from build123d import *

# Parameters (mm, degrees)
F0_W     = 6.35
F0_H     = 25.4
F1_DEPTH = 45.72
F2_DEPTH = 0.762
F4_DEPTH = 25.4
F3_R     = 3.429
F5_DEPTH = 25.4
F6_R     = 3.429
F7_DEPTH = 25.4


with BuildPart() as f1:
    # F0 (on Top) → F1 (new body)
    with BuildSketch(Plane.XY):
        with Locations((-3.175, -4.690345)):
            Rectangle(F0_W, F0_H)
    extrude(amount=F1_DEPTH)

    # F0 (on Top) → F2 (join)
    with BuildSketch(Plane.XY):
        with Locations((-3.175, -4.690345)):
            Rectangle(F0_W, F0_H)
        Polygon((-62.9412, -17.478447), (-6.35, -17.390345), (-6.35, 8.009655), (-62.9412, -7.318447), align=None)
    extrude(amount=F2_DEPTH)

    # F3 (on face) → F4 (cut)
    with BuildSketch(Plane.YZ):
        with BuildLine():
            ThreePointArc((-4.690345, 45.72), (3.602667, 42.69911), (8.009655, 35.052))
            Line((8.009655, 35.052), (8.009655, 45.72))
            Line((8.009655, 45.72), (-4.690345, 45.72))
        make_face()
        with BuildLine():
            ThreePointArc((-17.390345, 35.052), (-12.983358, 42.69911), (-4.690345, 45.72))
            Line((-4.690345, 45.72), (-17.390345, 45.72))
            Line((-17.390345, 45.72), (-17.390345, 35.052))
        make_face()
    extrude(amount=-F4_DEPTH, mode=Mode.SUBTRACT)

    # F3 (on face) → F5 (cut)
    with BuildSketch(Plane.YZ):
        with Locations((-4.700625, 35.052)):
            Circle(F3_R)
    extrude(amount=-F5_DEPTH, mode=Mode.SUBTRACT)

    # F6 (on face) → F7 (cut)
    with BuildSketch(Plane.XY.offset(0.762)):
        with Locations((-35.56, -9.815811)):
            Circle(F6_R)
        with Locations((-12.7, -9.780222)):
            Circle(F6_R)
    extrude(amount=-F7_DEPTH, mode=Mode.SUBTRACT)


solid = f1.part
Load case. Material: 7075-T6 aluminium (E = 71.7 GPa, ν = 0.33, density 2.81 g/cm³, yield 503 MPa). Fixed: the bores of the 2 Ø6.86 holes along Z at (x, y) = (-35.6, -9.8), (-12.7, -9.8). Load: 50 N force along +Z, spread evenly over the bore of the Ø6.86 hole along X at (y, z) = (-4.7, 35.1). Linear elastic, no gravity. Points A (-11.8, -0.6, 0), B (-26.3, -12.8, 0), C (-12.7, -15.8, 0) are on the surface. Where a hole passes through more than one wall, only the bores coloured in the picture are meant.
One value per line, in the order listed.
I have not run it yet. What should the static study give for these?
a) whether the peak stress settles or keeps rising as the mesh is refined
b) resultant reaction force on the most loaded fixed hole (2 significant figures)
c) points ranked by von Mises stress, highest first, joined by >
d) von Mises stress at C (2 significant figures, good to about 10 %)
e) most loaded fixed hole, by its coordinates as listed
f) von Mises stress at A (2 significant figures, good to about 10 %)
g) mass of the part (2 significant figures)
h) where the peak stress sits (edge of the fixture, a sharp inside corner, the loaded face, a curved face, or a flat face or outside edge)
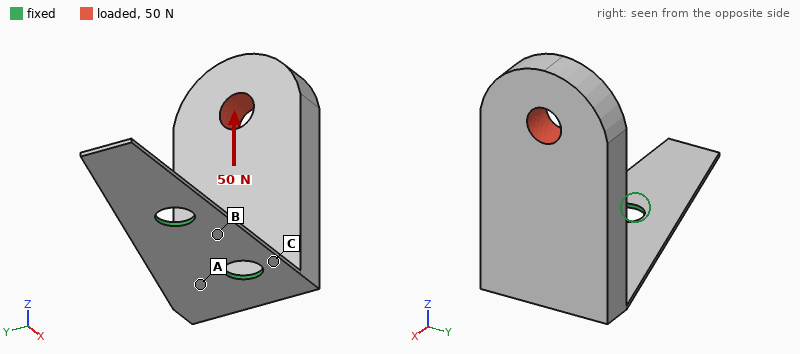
keeps rising
51 N
A > C > B
30 MPa
(-12.7, -9.8)
48 MPa
21 g
edge of the fixture
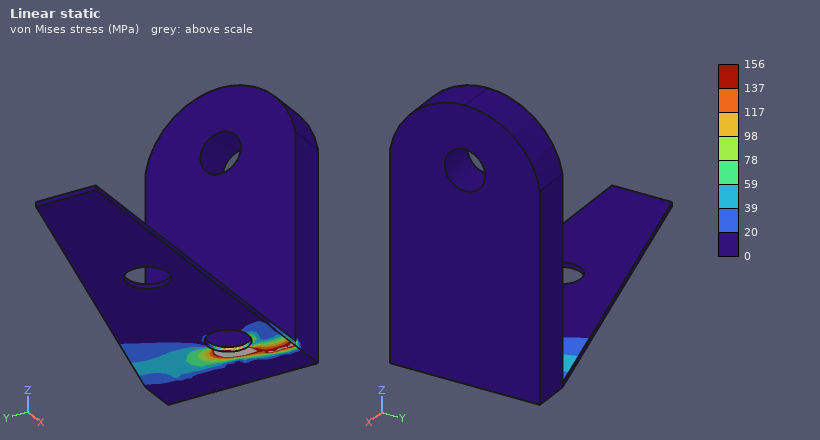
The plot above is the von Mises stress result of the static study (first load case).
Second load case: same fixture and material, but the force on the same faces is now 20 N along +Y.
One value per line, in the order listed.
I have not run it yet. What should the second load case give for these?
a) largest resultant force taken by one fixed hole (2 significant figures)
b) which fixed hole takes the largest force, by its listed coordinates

21 N
(-12.7, -9.8)
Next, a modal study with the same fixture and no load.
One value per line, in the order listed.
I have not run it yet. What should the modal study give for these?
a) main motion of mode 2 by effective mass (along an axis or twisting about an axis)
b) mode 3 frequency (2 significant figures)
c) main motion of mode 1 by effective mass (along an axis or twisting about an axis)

along Y
1200 Hz
along X
